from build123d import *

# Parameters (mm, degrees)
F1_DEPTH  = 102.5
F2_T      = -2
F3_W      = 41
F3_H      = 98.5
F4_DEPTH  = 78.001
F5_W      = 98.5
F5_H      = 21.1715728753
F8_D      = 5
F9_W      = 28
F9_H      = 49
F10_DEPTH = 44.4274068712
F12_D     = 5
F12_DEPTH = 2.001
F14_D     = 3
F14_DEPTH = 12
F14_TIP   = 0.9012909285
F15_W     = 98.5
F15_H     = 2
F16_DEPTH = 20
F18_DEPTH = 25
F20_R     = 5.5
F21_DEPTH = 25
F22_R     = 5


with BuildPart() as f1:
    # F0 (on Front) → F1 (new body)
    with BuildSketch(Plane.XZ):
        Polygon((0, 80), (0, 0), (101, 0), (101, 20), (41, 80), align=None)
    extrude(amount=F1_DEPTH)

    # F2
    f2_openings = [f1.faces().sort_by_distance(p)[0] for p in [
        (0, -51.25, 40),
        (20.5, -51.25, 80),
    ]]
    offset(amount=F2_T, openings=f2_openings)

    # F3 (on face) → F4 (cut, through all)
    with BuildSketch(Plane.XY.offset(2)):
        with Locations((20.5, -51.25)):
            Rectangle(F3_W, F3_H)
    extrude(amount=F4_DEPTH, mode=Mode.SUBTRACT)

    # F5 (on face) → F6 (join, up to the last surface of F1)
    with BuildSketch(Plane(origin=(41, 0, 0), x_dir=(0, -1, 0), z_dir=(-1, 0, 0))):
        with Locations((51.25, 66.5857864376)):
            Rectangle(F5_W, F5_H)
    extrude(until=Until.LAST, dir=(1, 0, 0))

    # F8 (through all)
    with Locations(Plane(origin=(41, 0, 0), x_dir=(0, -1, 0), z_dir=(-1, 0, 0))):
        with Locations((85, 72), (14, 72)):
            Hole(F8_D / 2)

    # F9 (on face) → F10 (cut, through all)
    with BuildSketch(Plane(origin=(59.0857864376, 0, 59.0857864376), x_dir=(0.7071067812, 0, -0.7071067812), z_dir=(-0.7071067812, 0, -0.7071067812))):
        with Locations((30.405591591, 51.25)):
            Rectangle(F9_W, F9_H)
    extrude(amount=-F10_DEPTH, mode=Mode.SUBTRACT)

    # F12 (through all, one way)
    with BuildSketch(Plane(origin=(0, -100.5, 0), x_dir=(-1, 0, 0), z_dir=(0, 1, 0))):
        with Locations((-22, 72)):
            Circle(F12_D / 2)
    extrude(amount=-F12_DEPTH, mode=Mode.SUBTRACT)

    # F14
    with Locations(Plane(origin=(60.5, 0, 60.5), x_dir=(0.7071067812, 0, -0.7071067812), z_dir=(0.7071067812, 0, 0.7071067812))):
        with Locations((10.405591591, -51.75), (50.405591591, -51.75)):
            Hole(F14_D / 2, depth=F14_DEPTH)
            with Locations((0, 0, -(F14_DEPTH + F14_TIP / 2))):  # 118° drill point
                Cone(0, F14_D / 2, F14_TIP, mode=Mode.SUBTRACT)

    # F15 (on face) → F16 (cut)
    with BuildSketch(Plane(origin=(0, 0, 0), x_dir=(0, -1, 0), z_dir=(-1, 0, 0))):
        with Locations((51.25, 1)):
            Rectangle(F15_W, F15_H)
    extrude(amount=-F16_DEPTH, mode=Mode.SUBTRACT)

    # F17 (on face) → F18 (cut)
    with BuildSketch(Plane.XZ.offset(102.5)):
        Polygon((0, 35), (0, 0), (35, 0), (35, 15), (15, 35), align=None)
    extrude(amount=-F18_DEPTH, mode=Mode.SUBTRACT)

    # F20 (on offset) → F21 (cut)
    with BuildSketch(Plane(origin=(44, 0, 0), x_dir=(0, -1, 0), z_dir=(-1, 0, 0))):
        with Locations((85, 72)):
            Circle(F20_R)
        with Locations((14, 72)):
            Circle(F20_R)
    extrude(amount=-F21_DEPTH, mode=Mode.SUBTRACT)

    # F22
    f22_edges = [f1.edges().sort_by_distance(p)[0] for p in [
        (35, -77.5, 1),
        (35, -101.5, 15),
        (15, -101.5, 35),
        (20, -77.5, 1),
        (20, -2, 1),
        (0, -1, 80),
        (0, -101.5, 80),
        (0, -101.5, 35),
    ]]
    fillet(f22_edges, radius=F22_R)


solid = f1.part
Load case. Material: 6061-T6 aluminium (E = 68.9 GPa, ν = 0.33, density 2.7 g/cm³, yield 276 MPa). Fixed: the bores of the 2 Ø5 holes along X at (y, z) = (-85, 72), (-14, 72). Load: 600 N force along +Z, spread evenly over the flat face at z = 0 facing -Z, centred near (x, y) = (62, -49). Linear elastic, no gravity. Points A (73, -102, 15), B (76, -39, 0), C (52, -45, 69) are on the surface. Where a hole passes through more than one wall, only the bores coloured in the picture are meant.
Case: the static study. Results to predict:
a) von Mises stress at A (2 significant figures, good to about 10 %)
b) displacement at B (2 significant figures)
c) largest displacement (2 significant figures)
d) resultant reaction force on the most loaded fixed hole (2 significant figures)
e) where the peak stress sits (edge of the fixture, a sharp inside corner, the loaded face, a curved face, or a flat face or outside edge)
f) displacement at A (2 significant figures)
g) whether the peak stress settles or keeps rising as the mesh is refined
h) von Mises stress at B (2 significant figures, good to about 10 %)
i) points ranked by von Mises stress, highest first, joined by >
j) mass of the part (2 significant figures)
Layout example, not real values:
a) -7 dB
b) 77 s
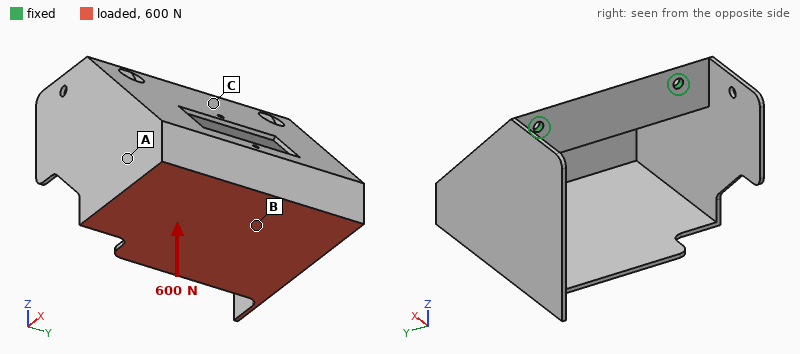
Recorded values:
a) 16 MPa
b) 0.39 mm
c) 0.81 mm
d) 310 N
e) edge of the fixture
f) 0.22 mm
g) keeps rising
h) 24 MPa
i) B > A > C
j) 210 g
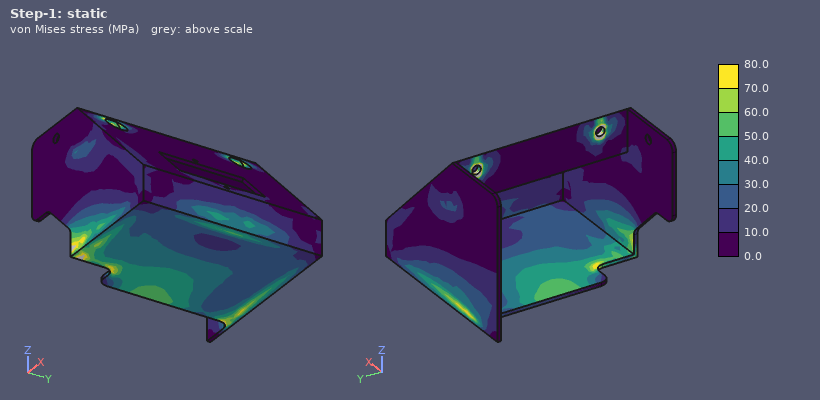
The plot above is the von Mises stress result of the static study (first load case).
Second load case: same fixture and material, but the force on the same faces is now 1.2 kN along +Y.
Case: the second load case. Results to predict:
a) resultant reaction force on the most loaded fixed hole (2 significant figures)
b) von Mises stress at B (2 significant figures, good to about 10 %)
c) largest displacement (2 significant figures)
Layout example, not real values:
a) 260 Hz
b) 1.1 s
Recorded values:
a) 1.3 kN
b) 18 MPa
c) 1.6 mm
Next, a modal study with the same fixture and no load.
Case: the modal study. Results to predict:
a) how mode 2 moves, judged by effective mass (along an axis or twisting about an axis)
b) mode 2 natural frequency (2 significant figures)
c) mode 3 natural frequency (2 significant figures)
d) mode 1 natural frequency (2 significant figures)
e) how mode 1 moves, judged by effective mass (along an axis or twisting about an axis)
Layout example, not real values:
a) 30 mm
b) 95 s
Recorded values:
a) along Y
b) 620 Hz
c) 850 Hz
d) 420 Hz
e) along X
